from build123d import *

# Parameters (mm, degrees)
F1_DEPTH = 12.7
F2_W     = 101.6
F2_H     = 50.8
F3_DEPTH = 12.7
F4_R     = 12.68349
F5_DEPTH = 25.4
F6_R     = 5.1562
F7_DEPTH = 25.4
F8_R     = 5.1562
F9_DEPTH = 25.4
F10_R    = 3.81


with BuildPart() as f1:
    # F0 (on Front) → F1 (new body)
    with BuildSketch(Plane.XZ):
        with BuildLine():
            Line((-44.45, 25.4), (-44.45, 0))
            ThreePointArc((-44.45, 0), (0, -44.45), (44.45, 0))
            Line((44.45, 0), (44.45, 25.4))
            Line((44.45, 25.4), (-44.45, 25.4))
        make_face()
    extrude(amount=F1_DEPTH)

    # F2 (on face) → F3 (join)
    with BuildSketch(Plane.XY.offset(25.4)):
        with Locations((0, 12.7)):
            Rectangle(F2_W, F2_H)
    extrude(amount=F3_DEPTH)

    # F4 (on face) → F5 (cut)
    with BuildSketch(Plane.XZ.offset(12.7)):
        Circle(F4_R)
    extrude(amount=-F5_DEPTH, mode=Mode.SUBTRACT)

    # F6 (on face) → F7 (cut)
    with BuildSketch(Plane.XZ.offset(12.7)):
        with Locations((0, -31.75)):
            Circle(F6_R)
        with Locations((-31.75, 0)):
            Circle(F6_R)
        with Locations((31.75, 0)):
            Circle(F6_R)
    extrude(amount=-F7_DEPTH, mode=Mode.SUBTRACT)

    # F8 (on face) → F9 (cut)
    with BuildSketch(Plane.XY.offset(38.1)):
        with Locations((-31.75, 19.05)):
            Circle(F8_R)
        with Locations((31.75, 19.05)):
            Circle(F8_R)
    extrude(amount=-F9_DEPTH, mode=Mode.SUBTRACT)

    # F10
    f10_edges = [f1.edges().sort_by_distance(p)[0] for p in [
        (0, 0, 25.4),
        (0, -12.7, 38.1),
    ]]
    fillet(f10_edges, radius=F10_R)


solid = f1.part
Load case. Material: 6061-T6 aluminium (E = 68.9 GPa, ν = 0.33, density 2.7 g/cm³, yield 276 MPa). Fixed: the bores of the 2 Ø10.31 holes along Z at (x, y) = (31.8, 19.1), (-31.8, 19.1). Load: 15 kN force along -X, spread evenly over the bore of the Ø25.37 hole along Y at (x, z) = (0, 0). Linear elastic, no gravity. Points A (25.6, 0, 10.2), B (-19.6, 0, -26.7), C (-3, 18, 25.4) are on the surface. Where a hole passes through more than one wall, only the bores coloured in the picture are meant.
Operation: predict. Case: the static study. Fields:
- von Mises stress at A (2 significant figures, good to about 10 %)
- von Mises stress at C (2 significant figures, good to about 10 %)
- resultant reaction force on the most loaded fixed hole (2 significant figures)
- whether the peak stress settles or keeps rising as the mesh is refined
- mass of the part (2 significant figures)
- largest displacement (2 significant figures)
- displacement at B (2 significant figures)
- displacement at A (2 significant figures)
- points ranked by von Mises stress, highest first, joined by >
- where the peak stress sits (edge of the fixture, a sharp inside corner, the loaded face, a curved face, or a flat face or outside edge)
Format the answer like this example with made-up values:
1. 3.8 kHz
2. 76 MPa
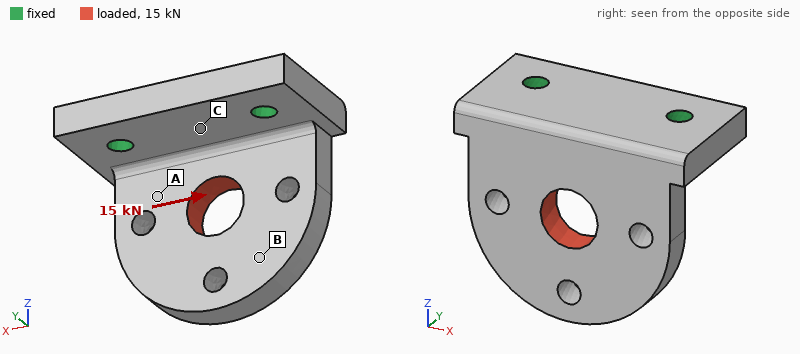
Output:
1. 48 MPa
2. 28 MPa
3. 11 kN
4. keeps rising
5. 330 g
6. 0.16 mm
7. 0.14 mm
8. 0.070 mm
9. A > C > B
10. edge of the fixture
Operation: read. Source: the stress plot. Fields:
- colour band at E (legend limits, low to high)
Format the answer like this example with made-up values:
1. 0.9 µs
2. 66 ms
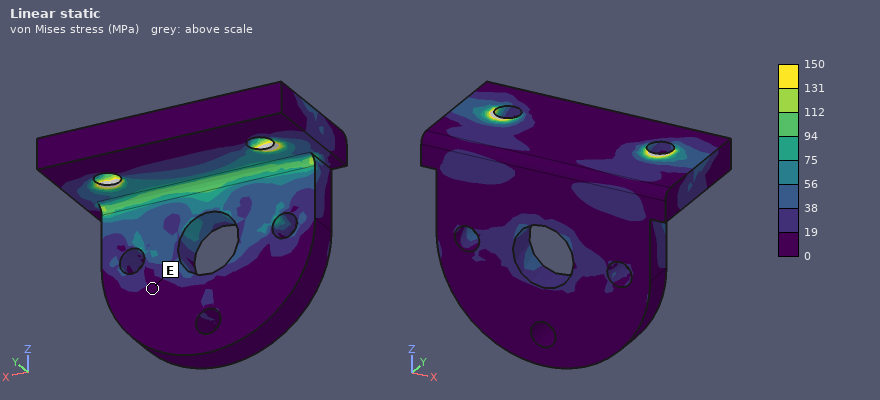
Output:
1. 0 to 19 MPa
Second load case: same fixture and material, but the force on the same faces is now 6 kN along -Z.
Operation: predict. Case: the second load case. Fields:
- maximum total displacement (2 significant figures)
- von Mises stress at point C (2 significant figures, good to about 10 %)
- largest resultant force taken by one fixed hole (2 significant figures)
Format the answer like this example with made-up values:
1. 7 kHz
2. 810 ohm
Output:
1. 0.15 mm
2. 15 MPa
3. 3.0 kN
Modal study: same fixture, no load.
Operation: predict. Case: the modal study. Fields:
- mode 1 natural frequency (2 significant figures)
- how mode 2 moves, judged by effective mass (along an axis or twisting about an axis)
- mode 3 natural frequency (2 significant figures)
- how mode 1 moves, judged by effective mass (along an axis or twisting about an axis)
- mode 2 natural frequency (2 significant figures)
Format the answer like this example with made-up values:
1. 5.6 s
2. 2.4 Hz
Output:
1. 1500 Hz
2. along X
3. 5000 Hz
4. along Y
5. 3500 Hz
